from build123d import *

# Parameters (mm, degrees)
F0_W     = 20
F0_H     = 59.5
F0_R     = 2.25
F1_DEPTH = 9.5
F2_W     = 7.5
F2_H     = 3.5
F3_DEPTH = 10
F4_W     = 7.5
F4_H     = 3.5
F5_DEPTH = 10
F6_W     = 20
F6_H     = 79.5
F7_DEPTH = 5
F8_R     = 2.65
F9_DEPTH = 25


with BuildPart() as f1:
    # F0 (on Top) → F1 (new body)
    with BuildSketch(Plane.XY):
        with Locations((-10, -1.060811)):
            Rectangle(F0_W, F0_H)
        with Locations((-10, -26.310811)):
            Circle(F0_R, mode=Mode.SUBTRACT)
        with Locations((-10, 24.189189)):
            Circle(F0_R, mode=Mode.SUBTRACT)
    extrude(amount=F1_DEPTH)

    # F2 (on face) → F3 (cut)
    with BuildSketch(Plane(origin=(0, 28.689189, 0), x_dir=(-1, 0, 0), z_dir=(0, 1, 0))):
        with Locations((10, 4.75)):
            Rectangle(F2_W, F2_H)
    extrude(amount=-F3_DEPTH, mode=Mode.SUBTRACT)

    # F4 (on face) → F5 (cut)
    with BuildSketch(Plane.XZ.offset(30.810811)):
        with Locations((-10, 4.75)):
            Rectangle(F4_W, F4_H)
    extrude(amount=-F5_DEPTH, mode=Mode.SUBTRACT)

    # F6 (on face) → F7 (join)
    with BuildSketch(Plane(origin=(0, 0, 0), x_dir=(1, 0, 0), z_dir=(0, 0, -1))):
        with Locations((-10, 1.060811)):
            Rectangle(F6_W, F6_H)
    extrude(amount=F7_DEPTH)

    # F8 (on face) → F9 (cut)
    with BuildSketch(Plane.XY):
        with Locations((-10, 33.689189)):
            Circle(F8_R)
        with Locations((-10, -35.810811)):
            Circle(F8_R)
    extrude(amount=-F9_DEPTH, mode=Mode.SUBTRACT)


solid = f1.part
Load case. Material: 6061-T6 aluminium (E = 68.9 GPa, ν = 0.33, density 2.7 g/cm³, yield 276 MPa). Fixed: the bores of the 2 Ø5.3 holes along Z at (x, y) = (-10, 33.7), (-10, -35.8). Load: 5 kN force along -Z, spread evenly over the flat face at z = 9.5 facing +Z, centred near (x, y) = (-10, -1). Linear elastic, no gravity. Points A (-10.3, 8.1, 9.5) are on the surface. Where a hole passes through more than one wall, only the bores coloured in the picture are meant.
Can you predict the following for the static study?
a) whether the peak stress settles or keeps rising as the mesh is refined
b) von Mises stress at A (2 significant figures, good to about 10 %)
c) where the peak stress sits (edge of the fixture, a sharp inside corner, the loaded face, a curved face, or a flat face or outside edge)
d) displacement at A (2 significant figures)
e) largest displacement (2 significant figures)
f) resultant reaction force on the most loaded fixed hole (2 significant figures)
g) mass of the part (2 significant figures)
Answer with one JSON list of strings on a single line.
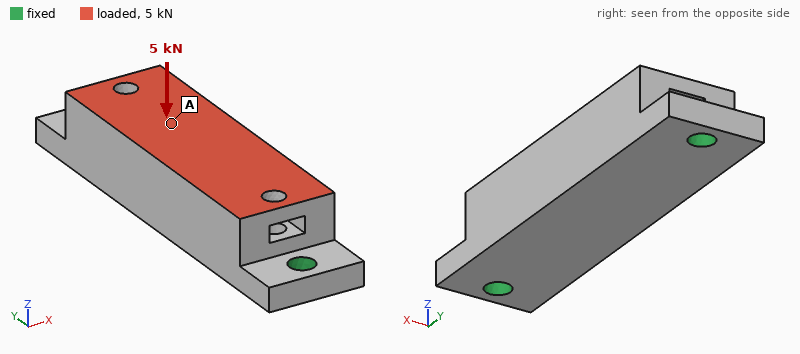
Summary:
["keeps rising", "37 MPa", "edge of the fixture", "43 µm", "48 µm", "3.4 kN", "49 g"]
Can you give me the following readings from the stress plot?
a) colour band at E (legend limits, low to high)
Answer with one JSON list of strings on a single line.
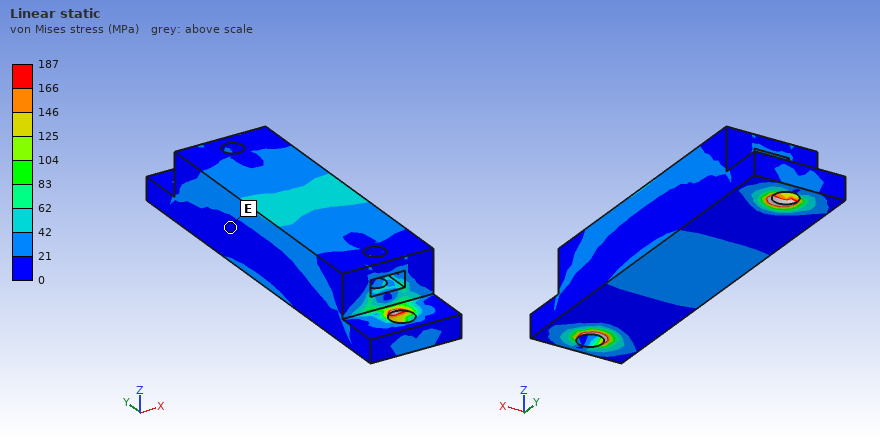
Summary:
["0 to 21 MPa"]
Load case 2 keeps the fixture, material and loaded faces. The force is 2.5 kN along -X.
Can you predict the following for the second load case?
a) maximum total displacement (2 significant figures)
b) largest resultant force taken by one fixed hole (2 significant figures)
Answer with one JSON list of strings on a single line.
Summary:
["86 µm", "1.3 kN"]
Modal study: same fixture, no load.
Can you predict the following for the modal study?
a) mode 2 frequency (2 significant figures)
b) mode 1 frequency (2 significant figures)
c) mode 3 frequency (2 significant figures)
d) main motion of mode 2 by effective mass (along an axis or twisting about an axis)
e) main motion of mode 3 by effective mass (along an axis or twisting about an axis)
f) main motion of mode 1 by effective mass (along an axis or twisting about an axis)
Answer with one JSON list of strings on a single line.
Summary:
["8400 Hz", "6500 Hz", "12 kHz", "along Z", "along X", "along X"]
